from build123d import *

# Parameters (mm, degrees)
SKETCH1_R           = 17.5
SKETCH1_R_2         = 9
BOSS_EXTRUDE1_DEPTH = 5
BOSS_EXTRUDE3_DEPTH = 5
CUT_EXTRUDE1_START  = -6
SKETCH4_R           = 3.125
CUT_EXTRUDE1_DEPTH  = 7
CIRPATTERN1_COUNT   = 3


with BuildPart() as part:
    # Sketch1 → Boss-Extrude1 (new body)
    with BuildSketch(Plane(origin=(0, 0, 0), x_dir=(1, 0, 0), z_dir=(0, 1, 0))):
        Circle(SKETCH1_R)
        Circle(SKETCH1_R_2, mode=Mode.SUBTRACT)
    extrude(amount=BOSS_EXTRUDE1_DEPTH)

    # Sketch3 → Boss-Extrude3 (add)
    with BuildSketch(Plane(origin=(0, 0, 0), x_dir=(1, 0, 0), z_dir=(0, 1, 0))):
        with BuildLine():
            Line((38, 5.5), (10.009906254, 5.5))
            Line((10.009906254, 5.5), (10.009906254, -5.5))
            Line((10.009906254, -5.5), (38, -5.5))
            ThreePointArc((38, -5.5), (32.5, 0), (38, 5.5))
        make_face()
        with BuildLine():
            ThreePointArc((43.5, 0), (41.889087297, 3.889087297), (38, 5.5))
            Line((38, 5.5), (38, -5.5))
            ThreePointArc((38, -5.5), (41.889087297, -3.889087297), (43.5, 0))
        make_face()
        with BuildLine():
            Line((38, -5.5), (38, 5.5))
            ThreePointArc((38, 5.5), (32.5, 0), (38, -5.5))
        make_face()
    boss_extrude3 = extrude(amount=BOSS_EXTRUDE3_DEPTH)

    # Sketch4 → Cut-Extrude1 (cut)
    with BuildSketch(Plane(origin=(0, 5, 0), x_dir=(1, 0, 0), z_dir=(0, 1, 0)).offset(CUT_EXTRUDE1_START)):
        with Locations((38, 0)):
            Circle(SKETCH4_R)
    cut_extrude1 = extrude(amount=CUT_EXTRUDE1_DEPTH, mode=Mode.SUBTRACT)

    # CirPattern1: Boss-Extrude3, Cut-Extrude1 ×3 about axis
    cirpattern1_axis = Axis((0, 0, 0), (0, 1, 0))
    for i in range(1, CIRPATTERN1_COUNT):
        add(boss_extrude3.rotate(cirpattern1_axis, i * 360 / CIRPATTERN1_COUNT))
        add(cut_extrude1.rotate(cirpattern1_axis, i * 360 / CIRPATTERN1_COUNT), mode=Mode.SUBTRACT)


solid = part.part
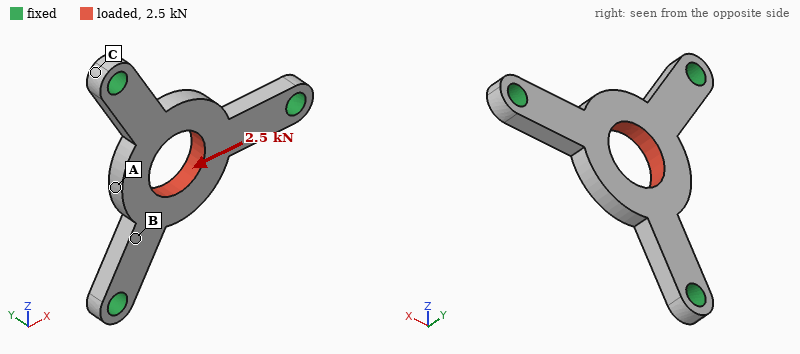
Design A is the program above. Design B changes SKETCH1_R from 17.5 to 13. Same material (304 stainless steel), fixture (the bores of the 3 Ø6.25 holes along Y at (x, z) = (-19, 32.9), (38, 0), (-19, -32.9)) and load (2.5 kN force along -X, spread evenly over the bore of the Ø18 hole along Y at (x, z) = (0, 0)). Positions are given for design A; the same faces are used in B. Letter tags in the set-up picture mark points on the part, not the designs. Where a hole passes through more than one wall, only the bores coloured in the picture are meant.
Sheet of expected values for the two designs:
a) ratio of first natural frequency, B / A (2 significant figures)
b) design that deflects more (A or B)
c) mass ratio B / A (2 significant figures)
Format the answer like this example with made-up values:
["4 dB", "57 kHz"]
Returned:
["1.1", "B", "0.81"]
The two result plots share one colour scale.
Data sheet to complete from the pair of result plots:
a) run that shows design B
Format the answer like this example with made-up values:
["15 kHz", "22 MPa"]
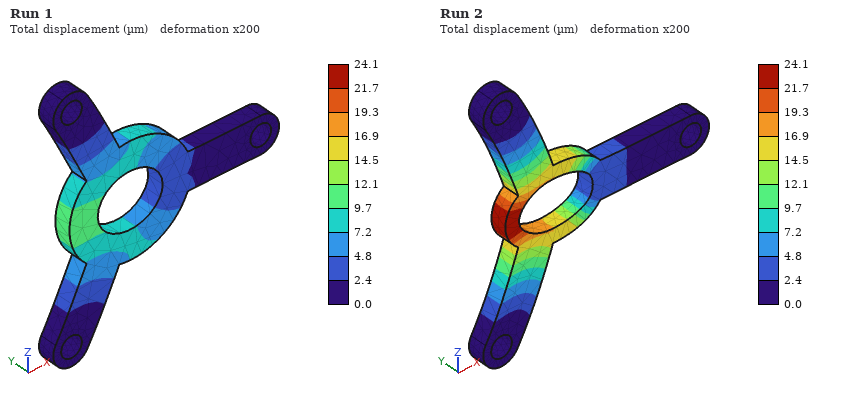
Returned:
["Run 2"]
